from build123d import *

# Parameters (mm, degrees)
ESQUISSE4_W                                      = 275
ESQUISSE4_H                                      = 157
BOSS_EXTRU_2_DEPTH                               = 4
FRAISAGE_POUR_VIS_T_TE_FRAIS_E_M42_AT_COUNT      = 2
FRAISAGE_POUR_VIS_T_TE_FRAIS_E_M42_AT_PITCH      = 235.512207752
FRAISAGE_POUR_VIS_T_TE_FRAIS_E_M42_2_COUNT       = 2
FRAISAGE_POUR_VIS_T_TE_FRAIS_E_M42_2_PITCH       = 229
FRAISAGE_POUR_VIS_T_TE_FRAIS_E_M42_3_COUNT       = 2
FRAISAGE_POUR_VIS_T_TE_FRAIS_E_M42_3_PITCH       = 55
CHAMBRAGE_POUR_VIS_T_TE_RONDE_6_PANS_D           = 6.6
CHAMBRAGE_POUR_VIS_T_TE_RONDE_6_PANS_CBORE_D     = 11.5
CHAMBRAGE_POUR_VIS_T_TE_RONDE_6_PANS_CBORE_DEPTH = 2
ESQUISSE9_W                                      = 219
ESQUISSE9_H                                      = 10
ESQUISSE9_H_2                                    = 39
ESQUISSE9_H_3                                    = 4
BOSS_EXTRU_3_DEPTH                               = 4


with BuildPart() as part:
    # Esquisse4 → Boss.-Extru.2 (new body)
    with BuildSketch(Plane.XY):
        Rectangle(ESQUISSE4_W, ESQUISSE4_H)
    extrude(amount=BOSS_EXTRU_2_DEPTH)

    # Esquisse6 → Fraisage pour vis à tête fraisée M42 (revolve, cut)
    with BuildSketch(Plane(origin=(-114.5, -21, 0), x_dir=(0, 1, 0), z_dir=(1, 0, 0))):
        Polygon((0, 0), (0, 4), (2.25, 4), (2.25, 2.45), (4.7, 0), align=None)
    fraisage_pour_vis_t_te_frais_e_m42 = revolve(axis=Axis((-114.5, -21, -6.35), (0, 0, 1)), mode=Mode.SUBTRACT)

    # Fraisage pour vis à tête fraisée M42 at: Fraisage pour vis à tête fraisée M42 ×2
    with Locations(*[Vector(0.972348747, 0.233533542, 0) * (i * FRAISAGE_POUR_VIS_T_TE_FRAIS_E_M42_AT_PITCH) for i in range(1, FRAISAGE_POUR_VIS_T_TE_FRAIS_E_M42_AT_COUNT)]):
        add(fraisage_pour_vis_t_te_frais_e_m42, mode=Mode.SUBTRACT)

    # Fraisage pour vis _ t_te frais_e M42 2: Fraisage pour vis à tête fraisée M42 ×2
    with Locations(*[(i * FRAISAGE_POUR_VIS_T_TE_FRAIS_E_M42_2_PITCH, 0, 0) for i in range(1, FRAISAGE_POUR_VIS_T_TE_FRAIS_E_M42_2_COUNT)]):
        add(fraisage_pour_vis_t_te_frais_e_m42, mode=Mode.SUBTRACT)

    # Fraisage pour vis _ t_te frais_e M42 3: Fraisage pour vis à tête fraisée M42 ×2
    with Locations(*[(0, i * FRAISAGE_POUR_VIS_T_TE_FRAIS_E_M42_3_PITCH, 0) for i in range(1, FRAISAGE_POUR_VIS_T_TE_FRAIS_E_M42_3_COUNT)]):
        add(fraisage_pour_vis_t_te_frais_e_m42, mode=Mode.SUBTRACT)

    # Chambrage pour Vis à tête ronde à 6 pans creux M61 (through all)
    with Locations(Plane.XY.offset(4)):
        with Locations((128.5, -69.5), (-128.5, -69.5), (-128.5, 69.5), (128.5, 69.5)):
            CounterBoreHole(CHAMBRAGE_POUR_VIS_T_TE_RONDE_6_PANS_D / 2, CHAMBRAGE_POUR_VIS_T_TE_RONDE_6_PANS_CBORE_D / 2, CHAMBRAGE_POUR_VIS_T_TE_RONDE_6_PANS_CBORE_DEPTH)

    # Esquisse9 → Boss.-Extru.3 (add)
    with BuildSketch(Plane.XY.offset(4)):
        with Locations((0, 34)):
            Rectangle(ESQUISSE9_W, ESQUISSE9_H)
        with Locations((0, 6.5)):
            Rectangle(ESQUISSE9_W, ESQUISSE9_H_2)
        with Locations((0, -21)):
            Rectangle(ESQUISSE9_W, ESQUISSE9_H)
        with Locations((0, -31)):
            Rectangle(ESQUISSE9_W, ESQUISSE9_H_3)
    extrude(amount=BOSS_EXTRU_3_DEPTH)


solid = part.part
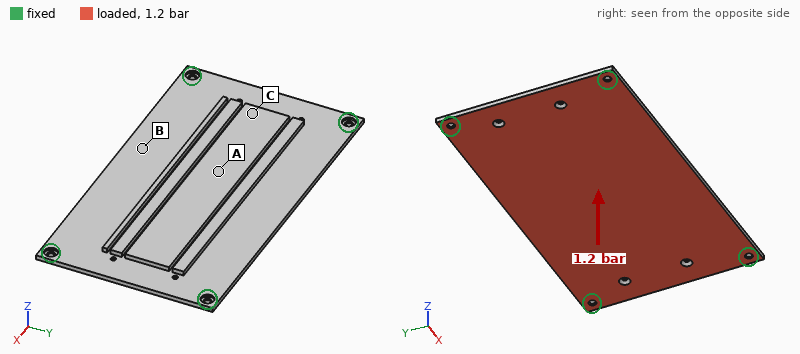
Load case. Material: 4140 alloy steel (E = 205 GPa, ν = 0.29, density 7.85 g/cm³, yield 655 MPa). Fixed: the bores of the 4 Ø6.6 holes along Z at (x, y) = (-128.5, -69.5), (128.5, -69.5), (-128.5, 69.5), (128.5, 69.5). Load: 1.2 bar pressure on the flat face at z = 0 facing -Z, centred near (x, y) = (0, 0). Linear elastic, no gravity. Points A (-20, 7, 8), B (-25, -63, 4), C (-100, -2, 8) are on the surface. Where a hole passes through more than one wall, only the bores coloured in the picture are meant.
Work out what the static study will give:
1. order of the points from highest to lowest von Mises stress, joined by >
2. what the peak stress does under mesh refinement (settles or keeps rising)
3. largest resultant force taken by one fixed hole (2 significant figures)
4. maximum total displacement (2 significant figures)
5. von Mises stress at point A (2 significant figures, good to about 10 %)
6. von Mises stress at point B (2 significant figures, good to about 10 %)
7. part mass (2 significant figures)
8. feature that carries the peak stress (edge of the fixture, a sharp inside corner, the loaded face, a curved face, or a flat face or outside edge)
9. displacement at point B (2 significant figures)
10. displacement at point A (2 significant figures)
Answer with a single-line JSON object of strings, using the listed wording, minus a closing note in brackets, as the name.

{"order of the points from highest to lowest von Mises stress, joined by >": "A > B > C", "what the peak stress does under mesh refinement": "keeps rising", "largest resultant force taken by one fixed hole": "5.8 kN", "maximum total displacement": "1.1 mm", "von Mises stress at point A": "110 MPa", "von Mises stress at point B": "68 MPa", "part mass": "1.8 kg", "feature that carries the peak stress": "edge of the fixture", "displacement at point B": "1.0 mm", "displacement at point A": "0.92 mm"}
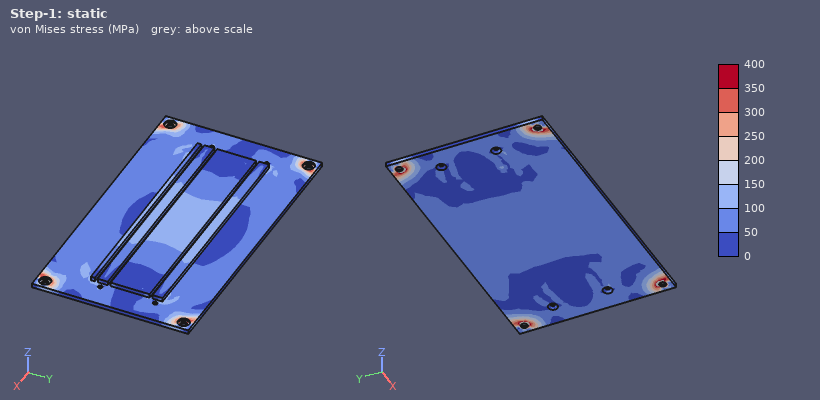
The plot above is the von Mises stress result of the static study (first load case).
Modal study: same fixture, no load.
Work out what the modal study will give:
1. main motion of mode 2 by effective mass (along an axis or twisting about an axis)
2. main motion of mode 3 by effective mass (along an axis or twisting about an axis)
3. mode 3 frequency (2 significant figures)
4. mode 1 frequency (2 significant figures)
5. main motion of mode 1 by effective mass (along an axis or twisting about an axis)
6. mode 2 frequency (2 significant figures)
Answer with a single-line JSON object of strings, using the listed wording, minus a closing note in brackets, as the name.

{"main motion of mode 2 by effective mass": "twisting about X", "main motion of mode 3 by effective mass": "twisting about Y", "mode 3 frequency": "740 Hz", "mode 1 frequency": "300 Hz", "main motion of mode 1 by effective mass": "along Z", "mode 2 frequency": "560 Hz"}
